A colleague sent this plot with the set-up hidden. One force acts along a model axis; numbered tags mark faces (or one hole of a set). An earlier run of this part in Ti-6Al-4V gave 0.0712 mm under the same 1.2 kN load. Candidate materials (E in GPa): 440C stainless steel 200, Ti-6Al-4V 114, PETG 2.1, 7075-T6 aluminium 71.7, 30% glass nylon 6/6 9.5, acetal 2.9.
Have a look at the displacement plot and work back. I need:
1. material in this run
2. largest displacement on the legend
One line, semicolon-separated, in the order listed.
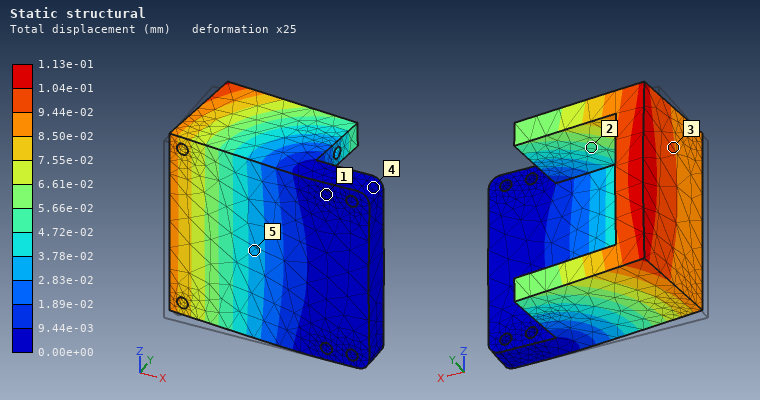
7075-T6 aluminium; 1.13e-01 mm
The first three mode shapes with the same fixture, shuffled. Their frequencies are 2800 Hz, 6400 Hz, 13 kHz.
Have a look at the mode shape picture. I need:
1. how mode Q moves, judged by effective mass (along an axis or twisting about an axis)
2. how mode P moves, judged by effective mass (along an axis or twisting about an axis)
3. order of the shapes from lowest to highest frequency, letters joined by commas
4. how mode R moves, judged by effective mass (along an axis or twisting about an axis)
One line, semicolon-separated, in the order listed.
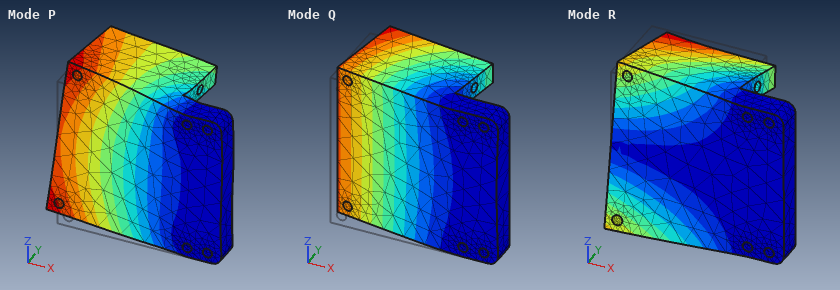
along Y; along Z; Q, R, P; along Z
